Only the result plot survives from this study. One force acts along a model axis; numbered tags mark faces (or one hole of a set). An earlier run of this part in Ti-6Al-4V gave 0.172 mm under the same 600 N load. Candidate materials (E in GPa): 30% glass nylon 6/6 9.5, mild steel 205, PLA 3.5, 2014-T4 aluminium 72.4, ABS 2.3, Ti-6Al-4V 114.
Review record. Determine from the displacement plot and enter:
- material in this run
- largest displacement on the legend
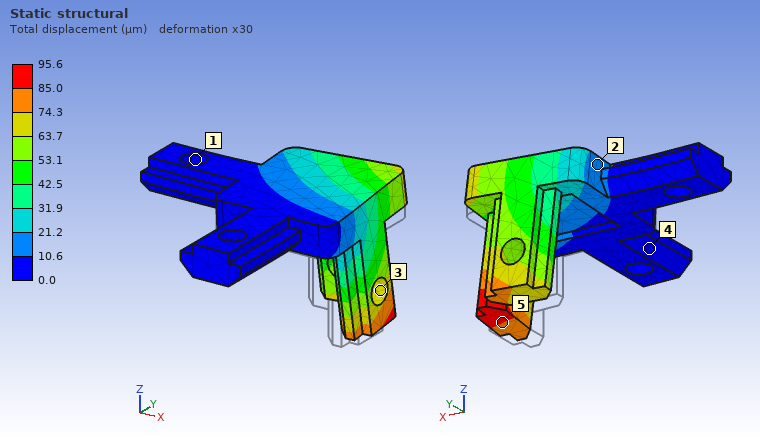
mild steel
95.6 µm
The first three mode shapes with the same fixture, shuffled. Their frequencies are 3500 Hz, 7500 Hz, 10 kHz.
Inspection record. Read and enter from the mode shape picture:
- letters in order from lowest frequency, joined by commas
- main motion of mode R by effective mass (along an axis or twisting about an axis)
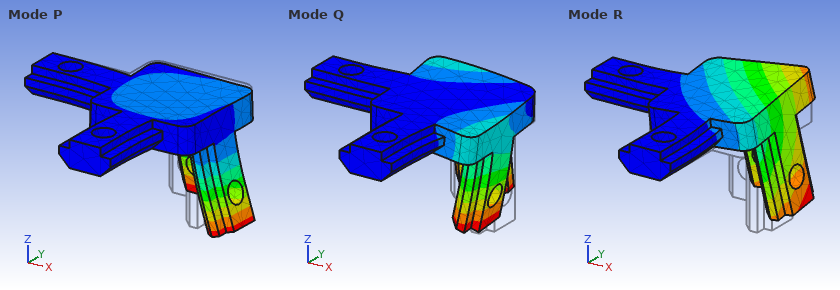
R, Q, P
along Z
